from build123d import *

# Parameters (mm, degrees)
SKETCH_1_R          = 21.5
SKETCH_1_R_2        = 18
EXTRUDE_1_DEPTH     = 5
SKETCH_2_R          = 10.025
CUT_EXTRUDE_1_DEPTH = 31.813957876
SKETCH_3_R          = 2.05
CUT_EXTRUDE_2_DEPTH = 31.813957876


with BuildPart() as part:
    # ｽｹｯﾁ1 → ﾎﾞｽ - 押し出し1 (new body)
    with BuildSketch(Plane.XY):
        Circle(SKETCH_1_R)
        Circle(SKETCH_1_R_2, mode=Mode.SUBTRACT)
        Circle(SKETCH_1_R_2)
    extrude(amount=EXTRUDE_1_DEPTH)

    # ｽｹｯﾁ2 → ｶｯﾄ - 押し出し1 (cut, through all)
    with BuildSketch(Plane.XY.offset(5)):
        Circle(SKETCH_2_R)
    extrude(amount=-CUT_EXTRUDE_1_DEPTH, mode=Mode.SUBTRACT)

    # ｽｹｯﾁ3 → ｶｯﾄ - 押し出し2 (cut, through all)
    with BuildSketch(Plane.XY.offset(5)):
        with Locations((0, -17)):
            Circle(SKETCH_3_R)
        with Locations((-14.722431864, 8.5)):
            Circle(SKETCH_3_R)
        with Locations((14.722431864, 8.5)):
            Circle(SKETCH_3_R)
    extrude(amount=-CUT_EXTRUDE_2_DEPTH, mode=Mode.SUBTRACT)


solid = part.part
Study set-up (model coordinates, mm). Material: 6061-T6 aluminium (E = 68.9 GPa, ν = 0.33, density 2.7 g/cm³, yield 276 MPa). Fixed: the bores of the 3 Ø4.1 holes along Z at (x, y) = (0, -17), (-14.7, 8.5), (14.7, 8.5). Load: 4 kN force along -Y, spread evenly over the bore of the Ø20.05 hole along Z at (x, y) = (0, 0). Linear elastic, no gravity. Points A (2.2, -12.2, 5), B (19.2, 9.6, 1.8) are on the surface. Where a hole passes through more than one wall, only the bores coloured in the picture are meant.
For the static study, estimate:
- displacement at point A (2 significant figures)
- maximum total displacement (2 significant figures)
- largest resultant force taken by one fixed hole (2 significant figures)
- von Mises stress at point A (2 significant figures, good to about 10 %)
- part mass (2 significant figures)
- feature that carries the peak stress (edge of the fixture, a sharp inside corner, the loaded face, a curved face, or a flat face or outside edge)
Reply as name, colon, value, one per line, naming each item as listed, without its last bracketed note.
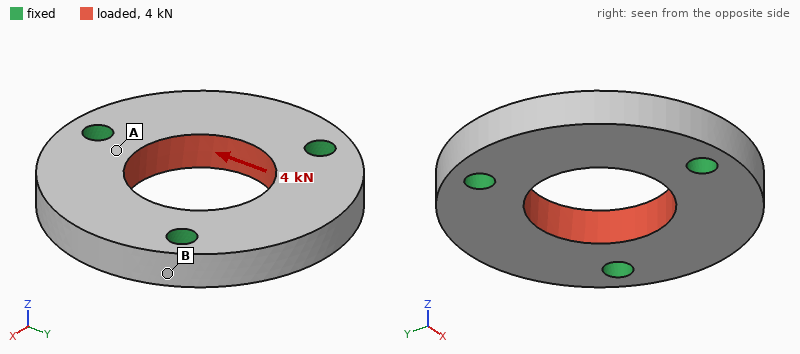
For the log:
displacement at point A: 1.3 µm
maximum total displacement: 6.9 µm
largest resultant force taken by one fixed hole: 1.5 kN
von Mises stress at point A: 23 MPa
part mass: 15 g
feature that carries the peak stress: edge of the fixture
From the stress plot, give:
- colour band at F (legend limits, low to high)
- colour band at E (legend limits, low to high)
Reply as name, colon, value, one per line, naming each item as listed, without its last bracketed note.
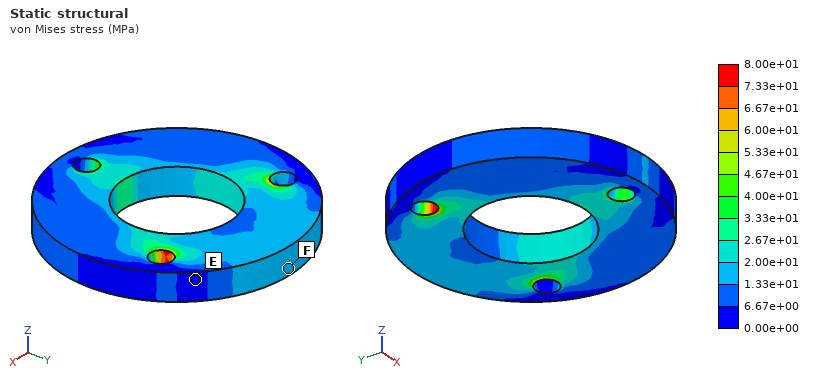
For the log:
colour band at F: 1.33e+01 to 2.00e+01 MPa
colour band at E: 0.00e+00 to 6.67e+00 MPa
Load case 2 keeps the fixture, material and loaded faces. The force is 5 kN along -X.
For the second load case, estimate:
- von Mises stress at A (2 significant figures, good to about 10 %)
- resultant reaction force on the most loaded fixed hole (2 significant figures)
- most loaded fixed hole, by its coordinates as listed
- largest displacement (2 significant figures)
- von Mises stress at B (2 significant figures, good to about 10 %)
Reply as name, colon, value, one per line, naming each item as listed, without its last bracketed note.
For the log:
von Mises stress at A: 28 MPa
resultant reaction force on the most loaded fixed hole: 2.0 kN
most loaded fixed hole, by its coordinates as listed: (0, -17)
largest displacement: 7.7 µm
von Mises stress at B: 15 MPa
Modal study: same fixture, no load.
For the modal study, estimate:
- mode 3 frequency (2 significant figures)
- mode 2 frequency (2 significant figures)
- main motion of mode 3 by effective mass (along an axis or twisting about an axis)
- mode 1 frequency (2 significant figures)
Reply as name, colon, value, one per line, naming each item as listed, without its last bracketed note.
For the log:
mode 3 frequency: 19 kHz
mode 2 frequency: 18 kHz
main motion of mode 3 by effective mass: along Z
mode 1 frequency: 18 kHz
